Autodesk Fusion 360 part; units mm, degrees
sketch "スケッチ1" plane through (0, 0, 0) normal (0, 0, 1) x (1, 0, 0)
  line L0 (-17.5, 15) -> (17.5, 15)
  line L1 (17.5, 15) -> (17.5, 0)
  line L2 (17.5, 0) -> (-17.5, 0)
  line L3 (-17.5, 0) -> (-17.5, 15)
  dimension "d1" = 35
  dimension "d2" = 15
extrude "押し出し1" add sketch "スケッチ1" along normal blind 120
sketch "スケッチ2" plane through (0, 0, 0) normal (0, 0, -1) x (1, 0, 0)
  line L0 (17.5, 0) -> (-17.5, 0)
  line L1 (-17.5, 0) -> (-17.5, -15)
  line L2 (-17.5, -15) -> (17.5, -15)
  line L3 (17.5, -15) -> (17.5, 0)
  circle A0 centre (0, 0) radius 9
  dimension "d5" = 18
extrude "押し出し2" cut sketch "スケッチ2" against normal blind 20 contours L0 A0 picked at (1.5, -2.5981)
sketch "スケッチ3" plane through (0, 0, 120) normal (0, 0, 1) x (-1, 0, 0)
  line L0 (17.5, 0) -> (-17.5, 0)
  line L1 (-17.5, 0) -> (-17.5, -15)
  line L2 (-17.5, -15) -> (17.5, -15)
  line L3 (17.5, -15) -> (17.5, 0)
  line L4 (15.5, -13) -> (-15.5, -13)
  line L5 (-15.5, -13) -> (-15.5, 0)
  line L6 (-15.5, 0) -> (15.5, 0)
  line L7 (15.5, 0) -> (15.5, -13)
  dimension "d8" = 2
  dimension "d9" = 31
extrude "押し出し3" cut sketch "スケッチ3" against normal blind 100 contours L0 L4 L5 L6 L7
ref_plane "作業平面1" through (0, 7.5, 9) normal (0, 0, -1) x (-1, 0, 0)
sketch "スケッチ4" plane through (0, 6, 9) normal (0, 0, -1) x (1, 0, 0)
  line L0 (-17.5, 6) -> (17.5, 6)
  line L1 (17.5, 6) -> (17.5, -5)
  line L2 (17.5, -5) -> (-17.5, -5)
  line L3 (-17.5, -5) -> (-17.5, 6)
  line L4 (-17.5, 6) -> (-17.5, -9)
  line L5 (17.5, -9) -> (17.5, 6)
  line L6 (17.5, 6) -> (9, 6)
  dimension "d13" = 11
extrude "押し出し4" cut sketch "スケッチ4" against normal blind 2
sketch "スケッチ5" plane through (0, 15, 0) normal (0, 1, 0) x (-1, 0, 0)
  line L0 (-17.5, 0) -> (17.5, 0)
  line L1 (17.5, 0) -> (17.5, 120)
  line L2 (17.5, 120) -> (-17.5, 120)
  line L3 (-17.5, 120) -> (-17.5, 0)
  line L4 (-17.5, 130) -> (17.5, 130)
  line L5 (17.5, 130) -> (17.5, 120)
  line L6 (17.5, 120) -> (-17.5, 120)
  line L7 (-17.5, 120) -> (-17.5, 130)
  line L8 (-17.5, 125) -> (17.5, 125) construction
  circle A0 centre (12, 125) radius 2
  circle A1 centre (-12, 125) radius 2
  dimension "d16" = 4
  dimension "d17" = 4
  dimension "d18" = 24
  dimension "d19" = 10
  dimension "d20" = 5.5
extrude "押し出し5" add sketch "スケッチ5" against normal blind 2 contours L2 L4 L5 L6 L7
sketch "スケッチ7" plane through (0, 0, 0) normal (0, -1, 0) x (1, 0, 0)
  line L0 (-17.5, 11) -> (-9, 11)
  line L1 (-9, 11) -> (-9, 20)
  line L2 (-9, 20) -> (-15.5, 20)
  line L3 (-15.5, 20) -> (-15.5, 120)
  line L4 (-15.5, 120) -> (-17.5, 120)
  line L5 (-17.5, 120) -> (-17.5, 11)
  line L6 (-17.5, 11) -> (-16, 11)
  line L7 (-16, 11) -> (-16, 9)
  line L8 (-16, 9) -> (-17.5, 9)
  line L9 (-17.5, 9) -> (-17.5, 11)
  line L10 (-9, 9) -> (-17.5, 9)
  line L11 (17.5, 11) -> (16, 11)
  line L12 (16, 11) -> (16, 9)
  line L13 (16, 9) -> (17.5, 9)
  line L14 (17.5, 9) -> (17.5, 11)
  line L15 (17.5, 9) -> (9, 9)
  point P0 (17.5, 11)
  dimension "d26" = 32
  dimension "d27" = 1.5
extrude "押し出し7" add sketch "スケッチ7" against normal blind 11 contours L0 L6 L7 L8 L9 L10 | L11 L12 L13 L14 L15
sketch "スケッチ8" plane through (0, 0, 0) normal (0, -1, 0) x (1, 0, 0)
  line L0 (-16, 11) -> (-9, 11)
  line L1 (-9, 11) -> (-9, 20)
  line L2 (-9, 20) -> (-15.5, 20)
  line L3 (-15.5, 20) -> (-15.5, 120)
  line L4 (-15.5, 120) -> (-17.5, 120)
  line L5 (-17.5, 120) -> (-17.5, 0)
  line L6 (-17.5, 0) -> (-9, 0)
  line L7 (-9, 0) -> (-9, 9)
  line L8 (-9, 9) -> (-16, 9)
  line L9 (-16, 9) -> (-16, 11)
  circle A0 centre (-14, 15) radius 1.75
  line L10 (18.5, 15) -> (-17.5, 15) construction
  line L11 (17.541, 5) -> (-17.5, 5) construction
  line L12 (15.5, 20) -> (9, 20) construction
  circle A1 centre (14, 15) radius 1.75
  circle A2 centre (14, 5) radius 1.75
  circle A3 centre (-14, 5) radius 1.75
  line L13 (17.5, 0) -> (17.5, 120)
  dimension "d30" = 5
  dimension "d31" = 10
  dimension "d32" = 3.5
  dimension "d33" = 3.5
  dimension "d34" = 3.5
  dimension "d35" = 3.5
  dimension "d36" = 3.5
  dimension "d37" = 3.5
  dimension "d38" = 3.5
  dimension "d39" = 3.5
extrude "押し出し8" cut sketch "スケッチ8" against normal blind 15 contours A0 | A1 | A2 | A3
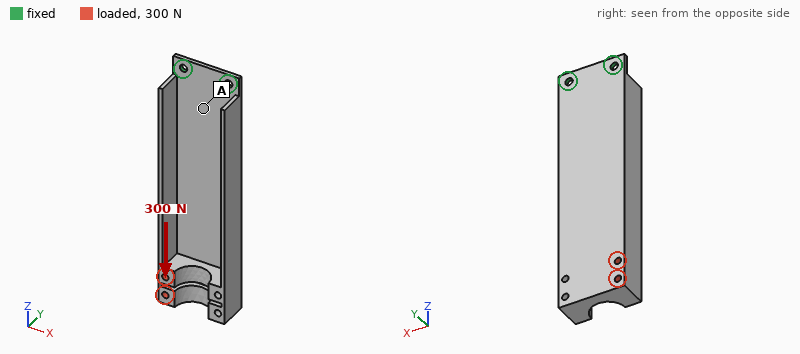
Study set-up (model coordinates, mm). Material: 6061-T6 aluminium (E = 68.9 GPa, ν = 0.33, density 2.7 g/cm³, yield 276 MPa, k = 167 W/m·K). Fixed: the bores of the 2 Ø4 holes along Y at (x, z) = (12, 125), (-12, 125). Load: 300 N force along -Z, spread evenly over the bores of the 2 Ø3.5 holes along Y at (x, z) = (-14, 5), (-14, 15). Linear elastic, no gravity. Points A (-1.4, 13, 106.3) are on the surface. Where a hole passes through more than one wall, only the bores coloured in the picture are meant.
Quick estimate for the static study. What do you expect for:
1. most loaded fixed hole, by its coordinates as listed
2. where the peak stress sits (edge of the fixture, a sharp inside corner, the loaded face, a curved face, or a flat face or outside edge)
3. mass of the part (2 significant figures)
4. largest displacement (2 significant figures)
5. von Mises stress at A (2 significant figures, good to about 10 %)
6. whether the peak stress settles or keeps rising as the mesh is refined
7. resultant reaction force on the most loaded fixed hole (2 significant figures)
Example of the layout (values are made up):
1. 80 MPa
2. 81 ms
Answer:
1. (-12, 125)
2. edge of the fixture
3. 53 g
4. 1.3 mm
5. 12 MPa
6. keeps rising
7. 320 N
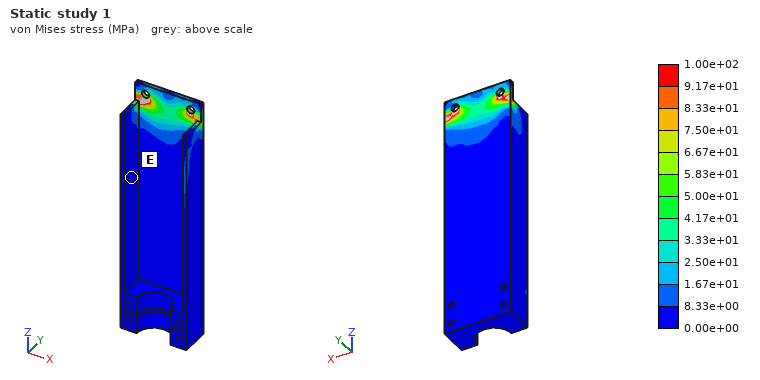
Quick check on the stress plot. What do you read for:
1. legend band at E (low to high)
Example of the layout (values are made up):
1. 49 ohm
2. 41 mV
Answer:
1. 0.00e+00 to 8.33e+00 MPa
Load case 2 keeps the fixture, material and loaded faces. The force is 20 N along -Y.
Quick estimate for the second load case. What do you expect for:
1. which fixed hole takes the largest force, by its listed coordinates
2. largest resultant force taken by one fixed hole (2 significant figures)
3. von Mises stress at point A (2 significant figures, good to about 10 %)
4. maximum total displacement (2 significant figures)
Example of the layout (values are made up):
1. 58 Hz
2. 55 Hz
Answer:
1. (-12, 125)
2. 41 N
3. 12 MPa
4. 1.5 mm
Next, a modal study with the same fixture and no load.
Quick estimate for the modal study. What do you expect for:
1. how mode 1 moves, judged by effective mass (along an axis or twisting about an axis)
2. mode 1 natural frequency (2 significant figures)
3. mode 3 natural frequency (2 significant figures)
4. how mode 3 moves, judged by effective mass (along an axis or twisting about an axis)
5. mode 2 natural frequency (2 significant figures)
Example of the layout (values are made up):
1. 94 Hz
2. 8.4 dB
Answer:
1. along Y
2. 120 Hz
3. 1100 Hz
4. along X
5. 650 Hz
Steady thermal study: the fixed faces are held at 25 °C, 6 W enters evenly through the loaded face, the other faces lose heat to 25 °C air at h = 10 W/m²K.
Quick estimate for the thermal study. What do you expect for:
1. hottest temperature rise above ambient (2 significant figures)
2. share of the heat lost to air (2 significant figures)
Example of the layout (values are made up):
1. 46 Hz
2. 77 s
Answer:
1. 27 K
2. 40 %
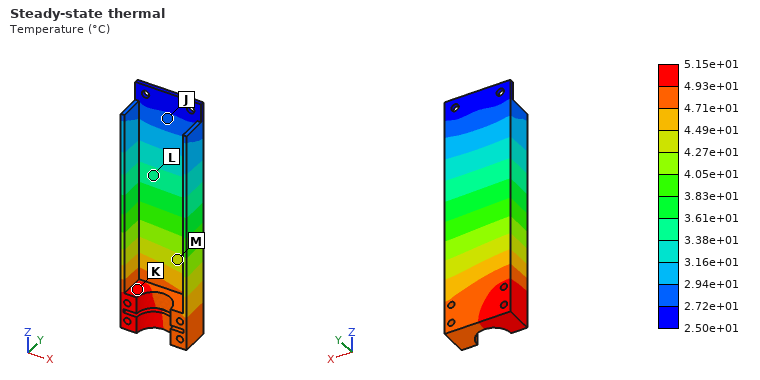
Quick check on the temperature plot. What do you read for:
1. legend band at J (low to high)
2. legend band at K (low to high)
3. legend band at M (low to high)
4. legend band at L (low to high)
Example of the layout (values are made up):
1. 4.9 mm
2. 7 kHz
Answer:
1. 2.72e+01 to 2.94e+01 °C
2. 4.93e+01 to 5.15e+01 °C
3. 4.27e+01 to 4.49e+01 °C
4. 3.38e+01 to 3.61e+01 °C
